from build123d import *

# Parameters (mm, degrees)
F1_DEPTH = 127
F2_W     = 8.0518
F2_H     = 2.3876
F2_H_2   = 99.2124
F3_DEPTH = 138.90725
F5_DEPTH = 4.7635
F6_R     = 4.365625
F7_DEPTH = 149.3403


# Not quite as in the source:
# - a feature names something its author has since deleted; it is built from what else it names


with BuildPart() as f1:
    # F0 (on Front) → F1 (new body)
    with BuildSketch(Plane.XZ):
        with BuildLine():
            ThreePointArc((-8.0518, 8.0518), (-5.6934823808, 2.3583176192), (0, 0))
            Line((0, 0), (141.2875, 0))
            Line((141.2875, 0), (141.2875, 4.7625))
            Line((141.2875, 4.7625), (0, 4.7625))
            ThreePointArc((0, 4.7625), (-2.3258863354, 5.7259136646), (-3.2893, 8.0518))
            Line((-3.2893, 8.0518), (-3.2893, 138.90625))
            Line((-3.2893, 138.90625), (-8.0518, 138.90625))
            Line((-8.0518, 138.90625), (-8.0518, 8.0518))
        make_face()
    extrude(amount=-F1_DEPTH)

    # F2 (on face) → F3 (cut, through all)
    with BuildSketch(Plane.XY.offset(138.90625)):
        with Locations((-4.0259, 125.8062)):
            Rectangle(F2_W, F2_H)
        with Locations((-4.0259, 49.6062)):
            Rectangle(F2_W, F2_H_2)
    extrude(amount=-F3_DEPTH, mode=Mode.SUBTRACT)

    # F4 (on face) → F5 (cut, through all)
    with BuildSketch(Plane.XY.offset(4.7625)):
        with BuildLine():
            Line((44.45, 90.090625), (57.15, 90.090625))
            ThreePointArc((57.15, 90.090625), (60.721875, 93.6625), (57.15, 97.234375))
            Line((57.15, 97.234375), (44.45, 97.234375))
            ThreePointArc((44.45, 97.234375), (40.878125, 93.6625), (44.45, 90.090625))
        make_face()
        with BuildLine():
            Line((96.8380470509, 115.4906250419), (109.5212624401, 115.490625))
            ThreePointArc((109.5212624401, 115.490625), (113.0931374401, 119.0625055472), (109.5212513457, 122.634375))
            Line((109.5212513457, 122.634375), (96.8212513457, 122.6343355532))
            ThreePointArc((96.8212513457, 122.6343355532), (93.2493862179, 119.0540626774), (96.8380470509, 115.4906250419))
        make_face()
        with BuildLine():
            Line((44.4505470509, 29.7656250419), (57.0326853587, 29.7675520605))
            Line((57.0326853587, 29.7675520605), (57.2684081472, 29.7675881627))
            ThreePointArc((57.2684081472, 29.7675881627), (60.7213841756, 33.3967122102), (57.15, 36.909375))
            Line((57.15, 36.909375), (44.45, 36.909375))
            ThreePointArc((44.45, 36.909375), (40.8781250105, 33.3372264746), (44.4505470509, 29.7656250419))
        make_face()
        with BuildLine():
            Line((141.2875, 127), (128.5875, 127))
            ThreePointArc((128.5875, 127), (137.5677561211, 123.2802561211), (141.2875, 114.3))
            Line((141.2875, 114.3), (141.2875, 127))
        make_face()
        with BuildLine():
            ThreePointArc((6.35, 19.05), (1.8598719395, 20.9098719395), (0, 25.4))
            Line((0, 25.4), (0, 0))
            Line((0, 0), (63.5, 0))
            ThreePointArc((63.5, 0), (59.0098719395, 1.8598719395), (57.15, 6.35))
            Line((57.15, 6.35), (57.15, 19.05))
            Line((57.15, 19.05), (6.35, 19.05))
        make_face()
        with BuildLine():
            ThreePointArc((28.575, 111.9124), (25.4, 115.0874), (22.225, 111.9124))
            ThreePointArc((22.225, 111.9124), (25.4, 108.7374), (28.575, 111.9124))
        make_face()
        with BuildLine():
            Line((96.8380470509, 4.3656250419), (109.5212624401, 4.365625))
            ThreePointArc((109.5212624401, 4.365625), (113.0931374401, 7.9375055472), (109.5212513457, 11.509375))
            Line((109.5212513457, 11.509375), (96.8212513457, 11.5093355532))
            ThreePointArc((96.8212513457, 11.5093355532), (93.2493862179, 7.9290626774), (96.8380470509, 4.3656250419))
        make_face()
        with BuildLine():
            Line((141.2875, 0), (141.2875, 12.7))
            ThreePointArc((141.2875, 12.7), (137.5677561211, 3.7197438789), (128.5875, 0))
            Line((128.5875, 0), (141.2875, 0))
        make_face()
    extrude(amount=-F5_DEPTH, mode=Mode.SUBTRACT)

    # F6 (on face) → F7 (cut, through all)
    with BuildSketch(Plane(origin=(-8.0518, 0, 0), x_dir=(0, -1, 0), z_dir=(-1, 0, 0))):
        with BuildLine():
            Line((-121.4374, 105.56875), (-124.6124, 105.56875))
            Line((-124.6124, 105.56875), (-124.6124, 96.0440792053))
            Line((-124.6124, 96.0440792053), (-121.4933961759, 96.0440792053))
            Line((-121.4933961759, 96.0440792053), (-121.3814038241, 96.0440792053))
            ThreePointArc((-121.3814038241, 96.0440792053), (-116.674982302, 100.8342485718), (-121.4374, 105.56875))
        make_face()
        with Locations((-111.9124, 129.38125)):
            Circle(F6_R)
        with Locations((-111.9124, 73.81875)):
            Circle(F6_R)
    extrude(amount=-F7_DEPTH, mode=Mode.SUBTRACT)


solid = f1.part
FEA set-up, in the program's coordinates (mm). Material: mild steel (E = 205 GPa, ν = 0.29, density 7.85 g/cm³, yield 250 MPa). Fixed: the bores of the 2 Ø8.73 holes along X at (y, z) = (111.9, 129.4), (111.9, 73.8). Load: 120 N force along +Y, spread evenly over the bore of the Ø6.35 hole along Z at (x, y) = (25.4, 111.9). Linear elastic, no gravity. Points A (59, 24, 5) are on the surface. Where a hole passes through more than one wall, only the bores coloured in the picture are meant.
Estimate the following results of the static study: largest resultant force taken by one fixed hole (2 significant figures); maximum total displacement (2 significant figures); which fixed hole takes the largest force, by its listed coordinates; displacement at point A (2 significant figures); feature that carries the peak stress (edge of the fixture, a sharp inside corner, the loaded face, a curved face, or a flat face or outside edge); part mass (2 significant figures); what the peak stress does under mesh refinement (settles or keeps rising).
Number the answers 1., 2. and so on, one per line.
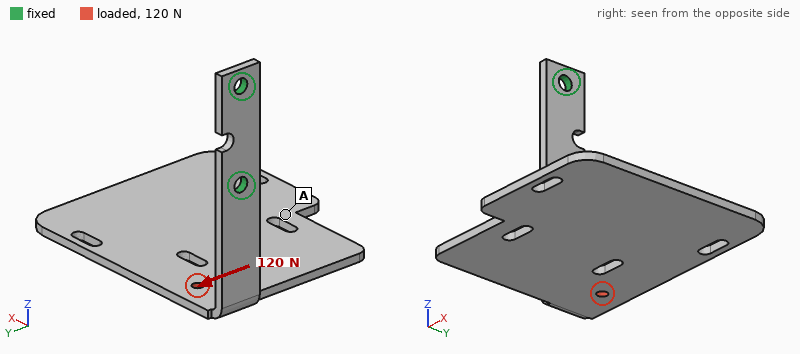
1. 190 N
2. 0.67 mm
3. (111.9, 73.8)
4. 0.41 mm
5. edge of the fixture
6. 730 g
7. keeps rising
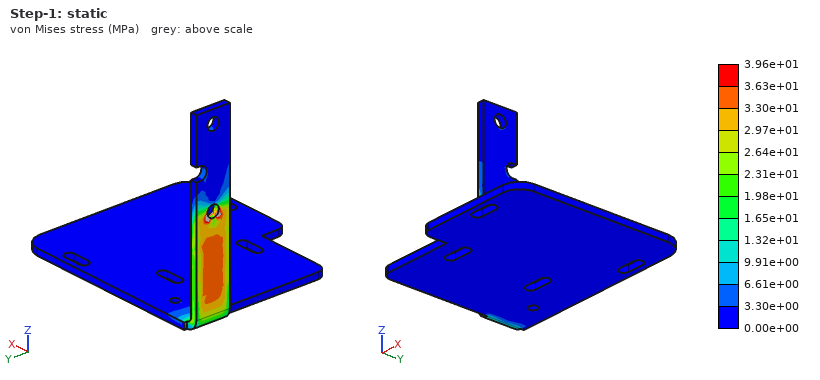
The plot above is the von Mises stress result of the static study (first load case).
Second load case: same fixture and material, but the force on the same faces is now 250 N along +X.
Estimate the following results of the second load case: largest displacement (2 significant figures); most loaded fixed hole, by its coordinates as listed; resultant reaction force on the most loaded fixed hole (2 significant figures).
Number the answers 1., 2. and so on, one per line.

1. 1.9 mm
2. (111.9, 73.8)
3. 250 N
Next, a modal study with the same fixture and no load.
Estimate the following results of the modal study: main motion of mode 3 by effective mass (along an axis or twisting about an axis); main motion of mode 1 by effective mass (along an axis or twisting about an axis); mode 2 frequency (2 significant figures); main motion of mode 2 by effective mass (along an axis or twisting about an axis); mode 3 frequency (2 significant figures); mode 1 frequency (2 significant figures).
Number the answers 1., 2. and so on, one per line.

1. along X
2. along Z
3. 63 Hz
4. along Y
5. 210 Hz
6. 49 Hz
